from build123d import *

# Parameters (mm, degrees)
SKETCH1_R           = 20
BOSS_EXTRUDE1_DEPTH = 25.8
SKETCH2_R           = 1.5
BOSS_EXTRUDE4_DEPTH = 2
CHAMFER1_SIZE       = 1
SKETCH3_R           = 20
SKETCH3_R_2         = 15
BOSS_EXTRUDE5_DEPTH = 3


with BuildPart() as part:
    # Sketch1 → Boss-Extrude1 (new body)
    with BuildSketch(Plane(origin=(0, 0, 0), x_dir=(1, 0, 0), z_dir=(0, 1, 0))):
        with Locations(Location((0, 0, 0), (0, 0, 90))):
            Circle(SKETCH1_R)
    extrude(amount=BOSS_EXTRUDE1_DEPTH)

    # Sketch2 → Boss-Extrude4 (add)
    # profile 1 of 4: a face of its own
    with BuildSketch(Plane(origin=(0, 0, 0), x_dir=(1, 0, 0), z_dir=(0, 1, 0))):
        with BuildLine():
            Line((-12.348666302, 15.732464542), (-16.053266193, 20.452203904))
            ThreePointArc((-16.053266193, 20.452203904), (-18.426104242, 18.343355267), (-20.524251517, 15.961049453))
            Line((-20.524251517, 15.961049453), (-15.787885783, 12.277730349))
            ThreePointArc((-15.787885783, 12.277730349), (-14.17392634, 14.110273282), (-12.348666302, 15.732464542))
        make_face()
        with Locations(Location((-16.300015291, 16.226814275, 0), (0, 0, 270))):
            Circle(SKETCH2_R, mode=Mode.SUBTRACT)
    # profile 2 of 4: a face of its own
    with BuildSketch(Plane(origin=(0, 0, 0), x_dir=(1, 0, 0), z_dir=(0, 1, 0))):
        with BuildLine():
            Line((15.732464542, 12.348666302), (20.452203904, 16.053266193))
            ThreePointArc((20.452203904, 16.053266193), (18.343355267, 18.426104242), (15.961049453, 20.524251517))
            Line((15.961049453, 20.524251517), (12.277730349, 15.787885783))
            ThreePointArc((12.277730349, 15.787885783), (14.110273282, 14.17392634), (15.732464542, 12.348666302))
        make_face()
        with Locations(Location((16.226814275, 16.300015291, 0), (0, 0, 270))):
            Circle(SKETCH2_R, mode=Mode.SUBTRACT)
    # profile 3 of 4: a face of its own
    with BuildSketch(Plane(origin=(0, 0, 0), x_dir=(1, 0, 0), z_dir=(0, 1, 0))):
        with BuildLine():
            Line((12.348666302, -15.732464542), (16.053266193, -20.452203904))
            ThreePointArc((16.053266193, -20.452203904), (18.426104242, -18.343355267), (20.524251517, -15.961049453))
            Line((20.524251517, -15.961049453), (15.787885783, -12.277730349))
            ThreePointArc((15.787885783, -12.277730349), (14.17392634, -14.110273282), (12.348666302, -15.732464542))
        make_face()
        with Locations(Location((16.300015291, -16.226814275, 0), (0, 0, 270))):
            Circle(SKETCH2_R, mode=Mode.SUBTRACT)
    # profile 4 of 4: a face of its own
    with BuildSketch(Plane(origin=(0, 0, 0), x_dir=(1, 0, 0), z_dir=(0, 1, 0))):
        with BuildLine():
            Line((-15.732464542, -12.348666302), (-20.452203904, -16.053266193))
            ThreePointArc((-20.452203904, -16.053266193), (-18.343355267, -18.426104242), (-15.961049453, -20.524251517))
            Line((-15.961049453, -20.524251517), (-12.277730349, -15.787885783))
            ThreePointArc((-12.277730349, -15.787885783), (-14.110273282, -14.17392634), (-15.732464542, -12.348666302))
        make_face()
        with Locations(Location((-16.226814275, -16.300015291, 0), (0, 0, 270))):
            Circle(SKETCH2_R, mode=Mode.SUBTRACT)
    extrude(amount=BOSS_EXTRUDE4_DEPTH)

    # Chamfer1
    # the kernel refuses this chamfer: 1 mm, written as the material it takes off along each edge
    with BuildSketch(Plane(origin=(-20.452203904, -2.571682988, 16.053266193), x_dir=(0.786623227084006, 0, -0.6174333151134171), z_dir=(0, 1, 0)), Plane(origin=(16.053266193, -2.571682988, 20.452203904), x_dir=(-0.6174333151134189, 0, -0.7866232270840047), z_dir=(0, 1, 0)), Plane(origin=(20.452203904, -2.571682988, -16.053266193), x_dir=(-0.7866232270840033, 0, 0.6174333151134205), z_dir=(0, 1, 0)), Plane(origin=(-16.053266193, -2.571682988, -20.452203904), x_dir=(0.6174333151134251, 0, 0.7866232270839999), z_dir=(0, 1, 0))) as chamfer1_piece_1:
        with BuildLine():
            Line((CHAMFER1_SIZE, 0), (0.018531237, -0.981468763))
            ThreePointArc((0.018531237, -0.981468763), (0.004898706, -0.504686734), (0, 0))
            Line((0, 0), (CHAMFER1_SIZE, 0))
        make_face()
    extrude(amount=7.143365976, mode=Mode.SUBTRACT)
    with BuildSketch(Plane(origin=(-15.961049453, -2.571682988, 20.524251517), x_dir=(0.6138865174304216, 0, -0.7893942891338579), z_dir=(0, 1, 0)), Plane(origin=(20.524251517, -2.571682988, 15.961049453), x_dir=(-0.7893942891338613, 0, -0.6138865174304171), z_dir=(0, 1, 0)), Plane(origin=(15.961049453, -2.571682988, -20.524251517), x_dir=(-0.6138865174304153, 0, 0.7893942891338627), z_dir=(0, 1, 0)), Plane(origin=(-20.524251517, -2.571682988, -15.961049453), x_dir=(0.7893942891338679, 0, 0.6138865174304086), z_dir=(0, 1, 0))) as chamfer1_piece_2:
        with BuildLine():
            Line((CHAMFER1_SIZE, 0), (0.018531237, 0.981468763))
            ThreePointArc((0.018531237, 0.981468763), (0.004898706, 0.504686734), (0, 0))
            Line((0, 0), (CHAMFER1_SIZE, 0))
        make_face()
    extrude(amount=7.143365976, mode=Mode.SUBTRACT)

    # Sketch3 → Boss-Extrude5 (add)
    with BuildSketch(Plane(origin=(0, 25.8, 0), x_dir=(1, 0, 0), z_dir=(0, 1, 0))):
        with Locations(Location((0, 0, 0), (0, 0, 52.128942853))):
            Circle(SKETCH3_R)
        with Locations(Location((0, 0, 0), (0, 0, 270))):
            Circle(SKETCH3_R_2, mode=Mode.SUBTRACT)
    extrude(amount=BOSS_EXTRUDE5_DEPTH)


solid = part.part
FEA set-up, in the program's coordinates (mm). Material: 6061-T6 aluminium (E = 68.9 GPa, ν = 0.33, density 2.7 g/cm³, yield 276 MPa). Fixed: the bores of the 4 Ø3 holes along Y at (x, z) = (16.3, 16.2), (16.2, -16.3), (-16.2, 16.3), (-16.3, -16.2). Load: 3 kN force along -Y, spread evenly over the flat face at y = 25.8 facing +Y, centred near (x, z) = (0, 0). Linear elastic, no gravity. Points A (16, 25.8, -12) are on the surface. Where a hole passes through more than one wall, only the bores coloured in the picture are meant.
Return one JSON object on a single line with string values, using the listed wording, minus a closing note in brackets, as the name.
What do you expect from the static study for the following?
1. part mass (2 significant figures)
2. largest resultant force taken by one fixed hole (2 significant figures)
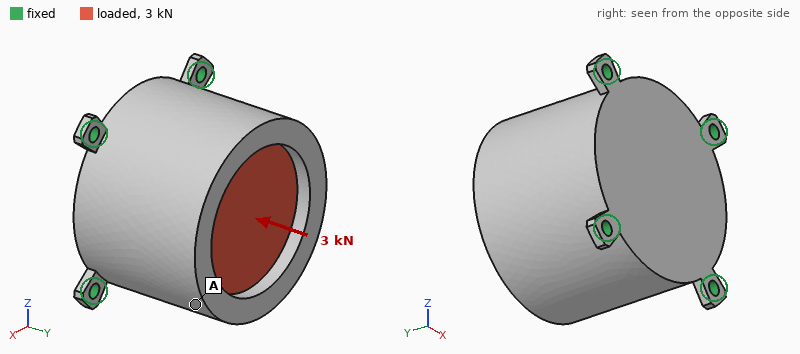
{"part mass": "93 g", "largest resultant force taken by one fixed hole": "840 N"}
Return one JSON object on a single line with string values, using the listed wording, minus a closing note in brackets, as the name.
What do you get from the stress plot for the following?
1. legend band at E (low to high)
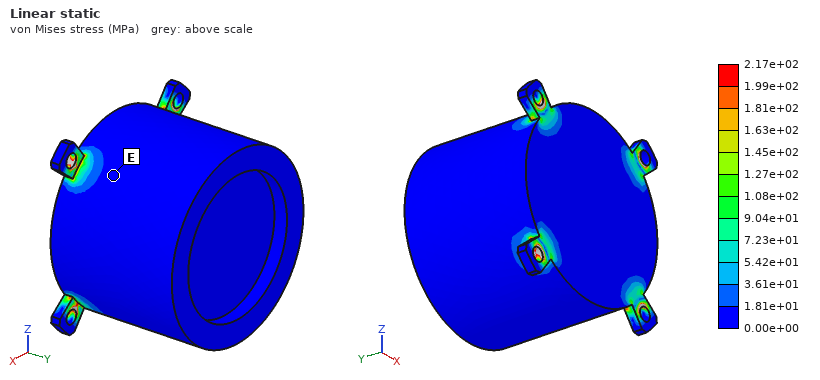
{"legend band at E": "0.00e+00 to 1.81e+01 MPa"}
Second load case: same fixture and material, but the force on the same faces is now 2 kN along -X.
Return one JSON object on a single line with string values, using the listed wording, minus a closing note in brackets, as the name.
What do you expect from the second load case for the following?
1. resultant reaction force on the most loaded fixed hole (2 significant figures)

{"resultant reaction force on the most loaded fixed hole": "1.1 kN"}
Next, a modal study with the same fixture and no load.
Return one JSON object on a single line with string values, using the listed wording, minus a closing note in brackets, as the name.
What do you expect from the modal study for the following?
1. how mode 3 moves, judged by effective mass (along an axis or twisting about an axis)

{"how mode 3 moves, judged by effective mass": "along Y"}
